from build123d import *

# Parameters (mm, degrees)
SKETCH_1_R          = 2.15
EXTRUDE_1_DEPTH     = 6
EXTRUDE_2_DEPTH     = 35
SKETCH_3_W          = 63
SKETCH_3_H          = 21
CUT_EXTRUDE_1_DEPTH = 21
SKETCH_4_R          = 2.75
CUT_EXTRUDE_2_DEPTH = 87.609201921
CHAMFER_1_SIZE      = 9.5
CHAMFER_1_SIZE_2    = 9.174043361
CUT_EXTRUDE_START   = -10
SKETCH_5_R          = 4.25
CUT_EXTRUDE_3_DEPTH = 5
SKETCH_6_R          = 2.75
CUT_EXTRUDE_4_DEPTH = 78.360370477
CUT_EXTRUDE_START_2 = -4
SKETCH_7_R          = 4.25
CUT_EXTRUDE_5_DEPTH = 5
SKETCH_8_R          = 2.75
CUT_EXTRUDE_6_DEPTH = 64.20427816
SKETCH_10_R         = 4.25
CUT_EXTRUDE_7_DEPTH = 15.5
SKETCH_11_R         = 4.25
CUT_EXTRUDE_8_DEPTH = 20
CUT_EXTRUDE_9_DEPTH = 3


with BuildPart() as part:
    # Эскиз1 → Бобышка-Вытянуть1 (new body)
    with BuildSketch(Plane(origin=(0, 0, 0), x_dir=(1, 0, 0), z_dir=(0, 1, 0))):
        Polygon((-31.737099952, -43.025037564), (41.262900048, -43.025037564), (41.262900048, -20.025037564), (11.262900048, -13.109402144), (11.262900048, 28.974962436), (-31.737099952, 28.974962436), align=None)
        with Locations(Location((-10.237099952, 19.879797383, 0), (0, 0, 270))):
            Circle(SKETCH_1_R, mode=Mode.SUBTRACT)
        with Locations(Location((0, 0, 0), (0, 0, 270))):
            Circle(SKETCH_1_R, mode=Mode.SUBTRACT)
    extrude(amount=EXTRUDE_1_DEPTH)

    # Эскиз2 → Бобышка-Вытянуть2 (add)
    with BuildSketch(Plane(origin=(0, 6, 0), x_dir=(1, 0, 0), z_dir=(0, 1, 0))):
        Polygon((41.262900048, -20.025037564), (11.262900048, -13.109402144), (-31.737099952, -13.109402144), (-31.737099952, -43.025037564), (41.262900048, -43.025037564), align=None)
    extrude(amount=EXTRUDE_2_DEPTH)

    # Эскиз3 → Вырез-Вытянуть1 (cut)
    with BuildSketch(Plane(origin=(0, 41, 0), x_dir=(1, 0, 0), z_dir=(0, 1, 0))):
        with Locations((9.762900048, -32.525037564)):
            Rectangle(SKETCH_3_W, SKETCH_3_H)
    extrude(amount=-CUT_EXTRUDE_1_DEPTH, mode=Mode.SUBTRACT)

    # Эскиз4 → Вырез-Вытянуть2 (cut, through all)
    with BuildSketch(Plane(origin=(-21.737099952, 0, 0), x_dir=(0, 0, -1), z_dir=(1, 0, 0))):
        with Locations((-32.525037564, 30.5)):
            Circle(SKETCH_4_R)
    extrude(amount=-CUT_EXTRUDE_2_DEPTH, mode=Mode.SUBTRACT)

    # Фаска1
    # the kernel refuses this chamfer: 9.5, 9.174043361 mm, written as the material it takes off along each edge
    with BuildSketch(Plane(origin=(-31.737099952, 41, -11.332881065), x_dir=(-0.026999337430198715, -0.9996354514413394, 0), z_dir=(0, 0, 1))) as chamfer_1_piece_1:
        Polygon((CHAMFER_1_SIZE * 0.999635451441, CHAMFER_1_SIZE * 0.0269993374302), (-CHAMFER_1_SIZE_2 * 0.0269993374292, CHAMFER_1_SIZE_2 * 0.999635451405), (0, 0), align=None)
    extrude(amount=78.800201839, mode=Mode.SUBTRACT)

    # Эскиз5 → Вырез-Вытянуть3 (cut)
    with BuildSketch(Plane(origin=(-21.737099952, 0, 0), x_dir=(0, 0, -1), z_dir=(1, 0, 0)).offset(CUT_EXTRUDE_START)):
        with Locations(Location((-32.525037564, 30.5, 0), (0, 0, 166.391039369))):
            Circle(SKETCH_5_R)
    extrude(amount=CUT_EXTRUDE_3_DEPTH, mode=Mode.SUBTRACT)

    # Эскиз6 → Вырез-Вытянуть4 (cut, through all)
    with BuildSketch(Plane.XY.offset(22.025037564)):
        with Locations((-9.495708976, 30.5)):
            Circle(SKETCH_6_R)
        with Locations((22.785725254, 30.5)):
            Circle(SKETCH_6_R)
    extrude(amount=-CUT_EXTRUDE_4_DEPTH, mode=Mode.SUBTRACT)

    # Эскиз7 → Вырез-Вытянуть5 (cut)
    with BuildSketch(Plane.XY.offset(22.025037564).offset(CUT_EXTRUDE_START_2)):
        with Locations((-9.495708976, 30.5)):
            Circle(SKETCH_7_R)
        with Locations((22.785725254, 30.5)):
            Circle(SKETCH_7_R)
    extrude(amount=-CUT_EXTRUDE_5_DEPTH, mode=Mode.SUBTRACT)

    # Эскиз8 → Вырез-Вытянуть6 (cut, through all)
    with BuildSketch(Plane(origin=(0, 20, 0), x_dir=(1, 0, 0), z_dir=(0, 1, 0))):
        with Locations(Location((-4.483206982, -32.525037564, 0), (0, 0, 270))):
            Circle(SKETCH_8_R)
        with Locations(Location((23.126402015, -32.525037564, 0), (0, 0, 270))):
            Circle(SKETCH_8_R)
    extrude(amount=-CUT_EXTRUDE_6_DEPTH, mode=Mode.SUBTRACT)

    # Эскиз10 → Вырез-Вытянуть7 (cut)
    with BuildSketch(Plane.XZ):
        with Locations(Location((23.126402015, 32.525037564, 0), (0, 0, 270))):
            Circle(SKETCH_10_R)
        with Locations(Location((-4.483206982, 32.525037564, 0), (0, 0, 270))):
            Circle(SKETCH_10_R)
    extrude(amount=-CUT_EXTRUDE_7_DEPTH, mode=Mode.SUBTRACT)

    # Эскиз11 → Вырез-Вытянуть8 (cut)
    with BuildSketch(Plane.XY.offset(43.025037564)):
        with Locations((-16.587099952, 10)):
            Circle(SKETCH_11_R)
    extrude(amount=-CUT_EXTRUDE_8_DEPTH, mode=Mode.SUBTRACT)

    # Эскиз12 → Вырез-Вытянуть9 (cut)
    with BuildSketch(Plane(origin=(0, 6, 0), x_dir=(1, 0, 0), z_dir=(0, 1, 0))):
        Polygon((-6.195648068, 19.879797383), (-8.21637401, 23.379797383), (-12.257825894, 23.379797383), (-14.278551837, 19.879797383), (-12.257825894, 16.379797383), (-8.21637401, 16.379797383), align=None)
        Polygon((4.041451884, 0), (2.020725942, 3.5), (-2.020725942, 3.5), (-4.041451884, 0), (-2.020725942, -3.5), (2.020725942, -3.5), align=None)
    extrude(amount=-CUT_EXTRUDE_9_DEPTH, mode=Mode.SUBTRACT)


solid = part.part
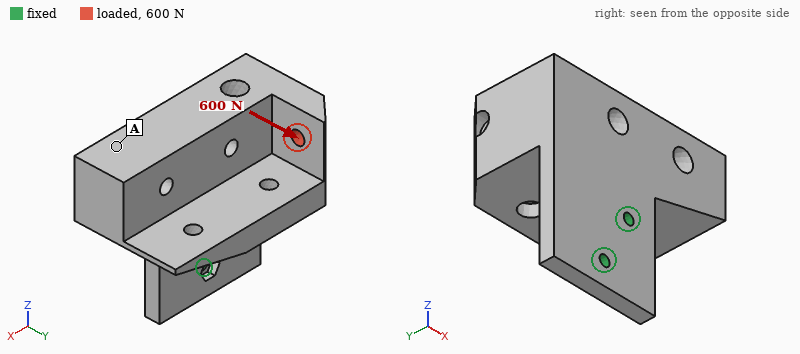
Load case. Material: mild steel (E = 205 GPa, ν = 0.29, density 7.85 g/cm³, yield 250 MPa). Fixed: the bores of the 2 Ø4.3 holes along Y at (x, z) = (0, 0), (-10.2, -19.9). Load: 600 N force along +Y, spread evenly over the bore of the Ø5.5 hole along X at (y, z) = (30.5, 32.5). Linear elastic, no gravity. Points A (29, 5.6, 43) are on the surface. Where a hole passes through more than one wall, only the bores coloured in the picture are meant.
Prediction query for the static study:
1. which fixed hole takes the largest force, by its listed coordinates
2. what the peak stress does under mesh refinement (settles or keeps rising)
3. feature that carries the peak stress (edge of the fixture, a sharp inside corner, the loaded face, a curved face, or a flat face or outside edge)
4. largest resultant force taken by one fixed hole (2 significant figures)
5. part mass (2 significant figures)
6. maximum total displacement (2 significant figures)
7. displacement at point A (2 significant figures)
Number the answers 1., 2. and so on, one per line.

1. (0, 0)
2. keeps rising
3. edge of the fixture
4. 970 N
5. 490 g
6. 0.22 mm
7. 0.054 mm
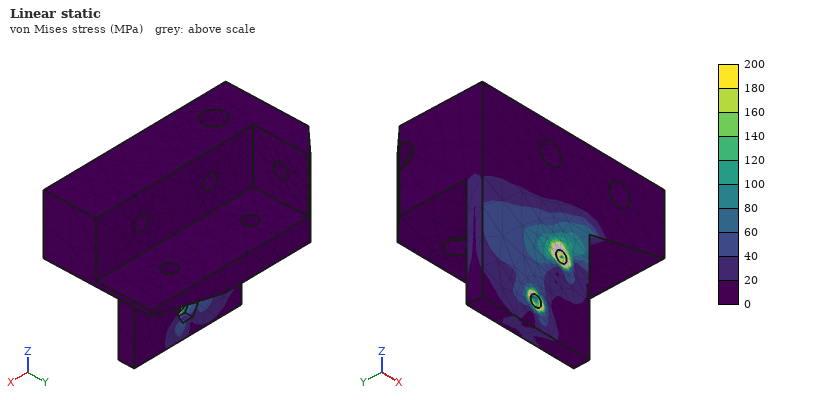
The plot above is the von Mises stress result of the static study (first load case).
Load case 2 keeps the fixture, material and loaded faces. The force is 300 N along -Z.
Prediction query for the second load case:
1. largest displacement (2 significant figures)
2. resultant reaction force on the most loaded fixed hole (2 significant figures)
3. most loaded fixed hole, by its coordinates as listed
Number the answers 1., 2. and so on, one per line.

1. 74 µm
2. 550 N
3. (-10.2, -19.9)
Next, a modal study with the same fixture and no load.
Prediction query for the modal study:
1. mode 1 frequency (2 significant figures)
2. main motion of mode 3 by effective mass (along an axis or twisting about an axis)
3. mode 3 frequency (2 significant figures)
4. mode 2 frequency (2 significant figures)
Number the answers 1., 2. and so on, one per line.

1. 680 Hz
2. along X
3. 2700 Hz
4. 910 Hz
